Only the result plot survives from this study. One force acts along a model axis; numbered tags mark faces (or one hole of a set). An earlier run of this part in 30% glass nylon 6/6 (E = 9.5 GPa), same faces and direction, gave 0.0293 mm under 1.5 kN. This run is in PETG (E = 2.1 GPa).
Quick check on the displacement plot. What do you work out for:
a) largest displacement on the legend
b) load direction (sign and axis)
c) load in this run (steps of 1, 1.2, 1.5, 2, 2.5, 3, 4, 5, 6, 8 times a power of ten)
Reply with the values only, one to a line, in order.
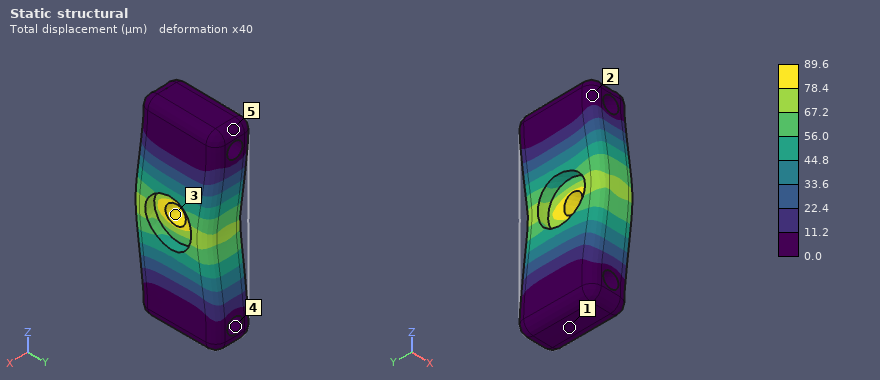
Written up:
89.6 µm
-Y
1 kN
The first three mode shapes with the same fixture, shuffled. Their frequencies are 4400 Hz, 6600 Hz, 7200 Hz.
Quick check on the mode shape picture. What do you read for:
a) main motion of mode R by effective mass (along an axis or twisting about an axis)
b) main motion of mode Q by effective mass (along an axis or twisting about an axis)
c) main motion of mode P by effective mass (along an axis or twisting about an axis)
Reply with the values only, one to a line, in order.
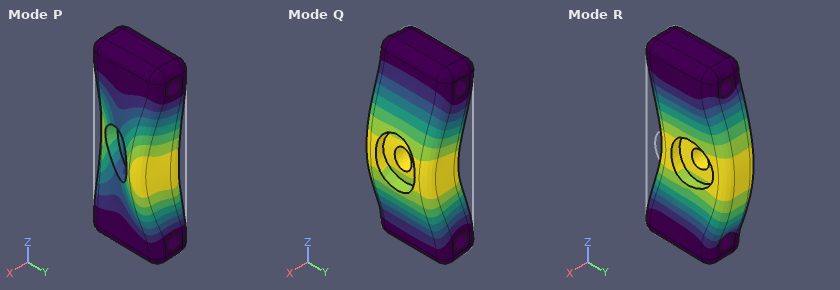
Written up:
along Y
along X
twisting about Z
